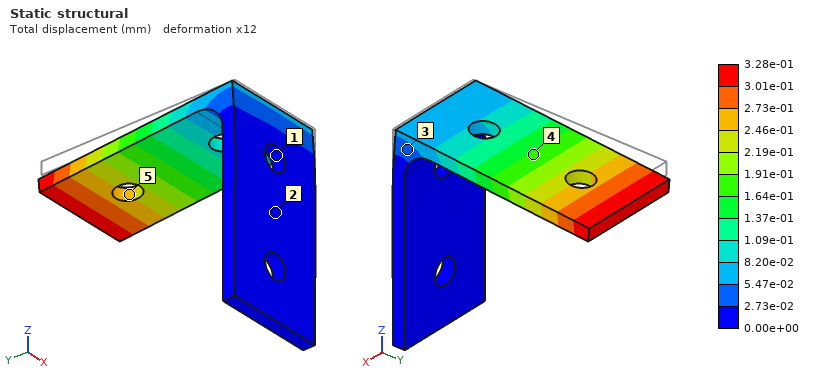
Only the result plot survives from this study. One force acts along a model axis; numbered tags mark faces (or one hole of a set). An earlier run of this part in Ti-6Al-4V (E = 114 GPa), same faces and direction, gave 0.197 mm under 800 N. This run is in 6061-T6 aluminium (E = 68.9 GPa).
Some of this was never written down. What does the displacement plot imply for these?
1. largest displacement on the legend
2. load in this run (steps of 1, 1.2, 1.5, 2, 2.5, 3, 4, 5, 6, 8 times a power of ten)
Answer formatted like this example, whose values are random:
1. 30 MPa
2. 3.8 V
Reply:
1. 3.28e-01 mm
2. 800 N
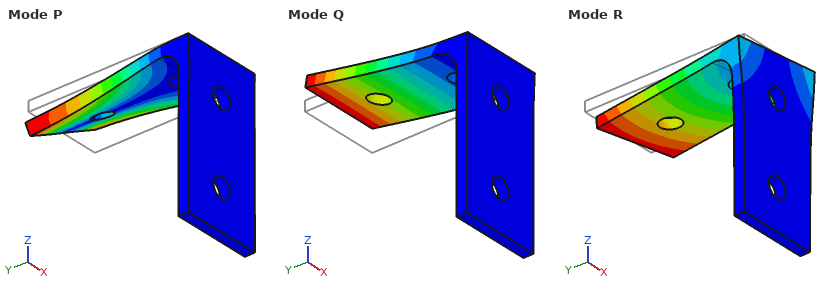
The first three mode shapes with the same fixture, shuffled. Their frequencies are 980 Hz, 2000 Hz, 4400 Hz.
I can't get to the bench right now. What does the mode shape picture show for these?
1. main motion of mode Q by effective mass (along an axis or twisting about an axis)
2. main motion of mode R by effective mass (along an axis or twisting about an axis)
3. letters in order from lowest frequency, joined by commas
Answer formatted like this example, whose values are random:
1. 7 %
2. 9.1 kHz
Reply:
1. along Z
2. along X
3. Q, R, P
